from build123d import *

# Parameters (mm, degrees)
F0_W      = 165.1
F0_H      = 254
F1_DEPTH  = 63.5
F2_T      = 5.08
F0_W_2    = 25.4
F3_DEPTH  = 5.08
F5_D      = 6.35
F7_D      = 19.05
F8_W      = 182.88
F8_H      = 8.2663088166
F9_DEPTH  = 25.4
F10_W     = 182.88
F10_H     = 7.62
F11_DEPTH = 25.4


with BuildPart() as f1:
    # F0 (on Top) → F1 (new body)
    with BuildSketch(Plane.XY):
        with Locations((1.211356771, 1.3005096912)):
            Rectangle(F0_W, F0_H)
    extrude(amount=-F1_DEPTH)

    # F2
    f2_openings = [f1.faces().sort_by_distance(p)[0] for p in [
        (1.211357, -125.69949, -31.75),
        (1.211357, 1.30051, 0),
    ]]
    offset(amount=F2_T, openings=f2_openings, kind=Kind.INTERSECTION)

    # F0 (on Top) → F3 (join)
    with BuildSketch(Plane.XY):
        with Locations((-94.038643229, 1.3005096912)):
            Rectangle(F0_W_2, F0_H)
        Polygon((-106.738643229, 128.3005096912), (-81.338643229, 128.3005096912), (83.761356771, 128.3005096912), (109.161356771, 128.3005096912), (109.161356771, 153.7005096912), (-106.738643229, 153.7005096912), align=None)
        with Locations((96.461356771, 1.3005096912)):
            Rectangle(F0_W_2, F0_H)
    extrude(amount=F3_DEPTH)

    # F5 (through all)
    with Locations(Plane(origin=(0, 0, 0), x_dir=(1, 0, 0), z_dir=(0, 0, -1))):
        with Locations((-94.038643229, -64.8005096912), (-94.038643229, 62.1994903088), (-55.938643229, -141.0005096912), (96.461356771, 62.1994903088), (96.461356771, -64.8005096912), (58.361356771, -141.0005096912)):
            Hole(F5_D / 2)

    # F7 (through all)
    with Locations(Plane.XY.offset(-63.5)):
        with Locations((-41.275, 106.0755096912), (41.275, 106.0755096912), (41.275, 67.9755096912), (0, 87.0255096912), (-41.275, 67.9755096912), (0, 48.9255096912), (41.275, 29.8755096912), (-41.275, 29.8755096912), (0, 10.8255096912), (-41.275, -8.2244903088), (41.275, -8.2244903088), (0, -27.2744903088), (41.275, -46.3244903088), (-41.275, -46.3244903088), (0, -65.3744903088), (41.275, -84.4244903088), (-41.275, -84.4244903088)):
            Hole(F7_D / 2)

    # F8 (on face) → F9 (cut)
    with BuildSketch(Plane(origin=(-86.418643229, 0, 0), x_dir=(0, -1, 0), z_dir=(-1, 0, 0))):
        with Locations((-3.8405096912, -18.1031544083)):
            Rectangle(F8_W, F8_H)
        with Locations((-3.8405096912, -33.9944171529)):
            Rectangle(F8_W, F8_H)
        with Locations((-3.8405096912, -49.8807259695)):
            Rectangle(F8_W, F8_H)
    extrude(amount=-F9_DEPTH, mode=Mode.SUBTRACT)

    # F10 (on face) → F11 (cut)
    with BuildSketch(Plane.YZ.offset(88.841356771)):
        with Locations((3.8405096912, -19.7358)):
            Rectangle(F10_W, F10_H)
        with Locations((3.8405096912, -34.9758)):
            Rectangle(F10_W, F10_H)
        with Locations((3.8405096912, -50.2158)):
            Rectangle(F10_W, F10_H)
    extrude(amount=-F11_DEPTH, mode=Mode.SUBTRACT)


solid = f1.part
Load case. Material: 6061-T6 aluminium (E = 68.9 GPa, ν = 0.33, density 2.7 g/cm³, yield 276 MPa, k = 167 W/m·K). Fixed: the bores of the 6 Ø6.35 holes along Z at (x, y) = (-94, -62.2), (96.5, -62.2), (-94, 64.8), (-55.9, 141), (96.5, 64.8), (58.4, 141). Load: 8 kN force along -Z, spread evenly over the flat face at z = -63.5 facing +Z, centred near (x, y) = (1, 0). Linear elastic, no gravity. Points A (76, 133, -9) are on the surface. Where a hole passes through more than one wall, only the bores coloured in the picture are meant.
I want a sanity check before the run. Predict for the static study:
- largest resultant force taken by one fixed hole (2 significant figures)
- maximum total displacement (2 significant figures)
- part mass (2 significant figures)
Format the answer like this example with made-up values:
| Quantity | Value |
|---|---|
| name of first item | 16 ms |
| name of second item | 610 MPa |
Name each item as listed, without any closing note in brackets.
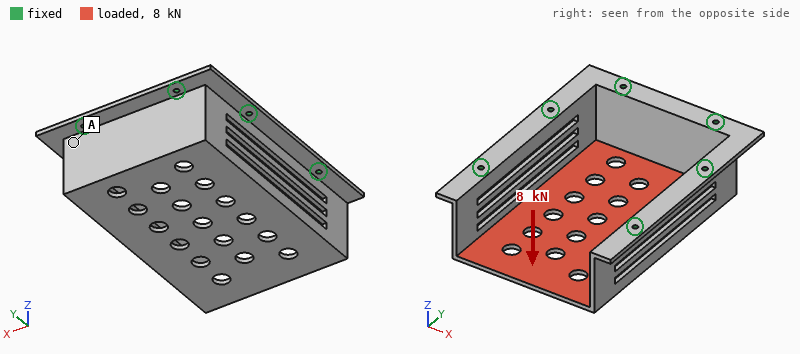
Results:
| Quantity | Value |
|---|---|
| largest resultant force taken by one fixed hole | 2.7 kN |
| maximum total displacement | 2.1 mm |
| part mass | 1.3 kg |
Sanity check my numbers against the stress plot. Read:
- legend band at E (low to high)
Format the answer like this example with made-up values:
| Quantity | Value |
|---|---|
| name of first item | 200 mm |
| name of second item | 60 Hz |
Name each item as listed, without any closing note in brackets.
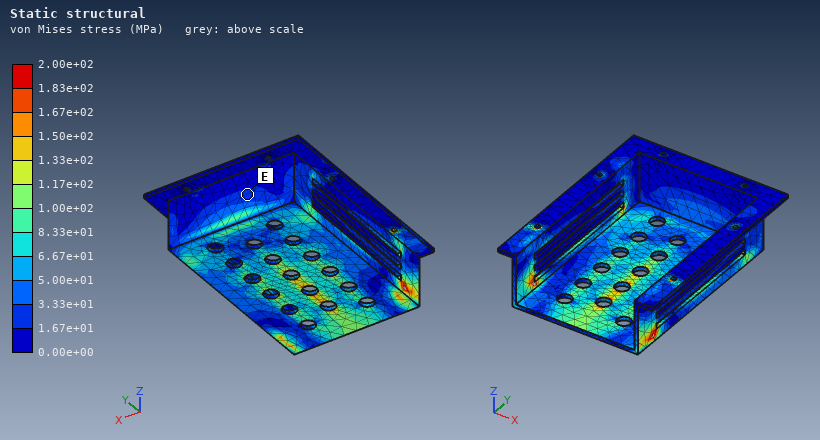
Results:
| Quantity | Value |
|---|---|
| legend band at E | 1.67e+01 to 3.33e+01 MPa |
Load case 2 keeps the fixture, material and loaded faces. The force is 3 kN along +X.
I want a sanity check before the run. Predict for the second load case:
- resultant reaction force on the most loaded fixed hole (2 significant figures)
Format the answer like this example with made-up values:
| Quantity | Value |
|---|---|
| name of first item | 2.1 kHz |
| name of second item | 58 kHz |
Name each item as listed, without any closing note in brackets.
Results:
| Quantity | Value |
|---|---|
| resultant reaction force on the most loaded fixed hole | 3.2 kN |
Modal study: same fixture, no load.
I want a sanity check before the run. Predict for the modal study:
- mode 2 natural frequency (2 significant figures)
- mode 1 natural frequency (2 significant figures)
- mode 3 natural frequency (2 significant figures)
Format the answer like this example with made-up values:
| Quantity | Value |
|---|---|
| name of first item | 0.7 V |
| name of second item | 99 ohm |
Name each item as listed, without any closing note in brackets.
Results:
| Quantity | Value |
|---|---|
| mode 2 natural frequency | 530 Hz |
| mode 1 natural frequency | 520 Hz |
| mode 3 natural frequency | 650 Hz |
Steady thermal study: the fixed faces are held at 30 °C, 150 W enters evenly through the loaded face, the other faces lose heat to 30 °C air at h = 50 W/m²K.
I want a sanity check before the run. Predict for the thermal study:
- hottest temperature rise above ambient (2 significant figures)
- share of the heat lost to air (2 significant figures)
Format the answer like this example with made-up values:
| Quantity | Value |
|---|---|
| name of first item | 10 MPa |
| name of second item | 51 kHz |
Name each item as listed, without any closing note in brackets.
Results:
| Quantity | Value |
|---|---|
| hottest temperature rise above ambient | 35 K |
| share of the heat lost to air | 77 % |
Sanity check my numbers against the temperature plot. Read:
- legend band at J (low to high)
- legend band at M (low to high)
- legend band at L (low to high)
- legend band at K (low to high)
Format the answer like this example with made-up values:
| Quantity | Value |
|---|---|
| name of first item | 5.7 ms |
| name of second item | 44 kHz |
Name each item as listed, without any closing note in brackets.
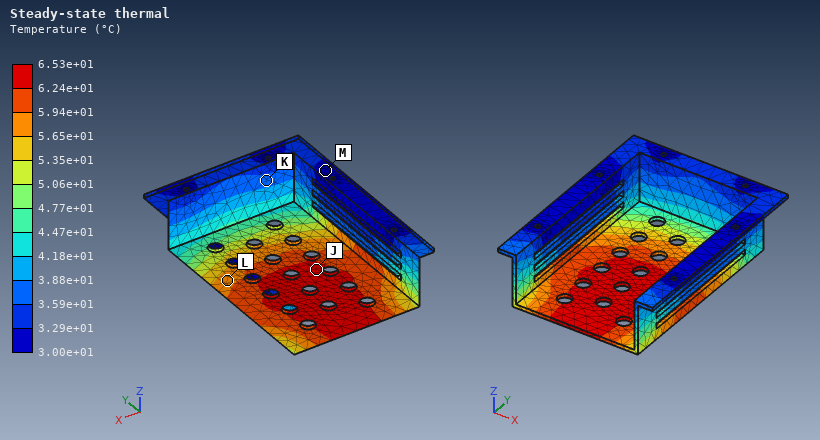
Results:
| Quantity | Value |
|---|---|
| legend band at J | 6.24e+01 to 6.53e+01 °C |
| legend band at M | 3.00e+01 to 3.29e+01 °C |
| legend band at L | 5.65e+01 to 5.94e+01 °C |
| legend band at K | 3.59e+01 to 3.88e+01 °C |
